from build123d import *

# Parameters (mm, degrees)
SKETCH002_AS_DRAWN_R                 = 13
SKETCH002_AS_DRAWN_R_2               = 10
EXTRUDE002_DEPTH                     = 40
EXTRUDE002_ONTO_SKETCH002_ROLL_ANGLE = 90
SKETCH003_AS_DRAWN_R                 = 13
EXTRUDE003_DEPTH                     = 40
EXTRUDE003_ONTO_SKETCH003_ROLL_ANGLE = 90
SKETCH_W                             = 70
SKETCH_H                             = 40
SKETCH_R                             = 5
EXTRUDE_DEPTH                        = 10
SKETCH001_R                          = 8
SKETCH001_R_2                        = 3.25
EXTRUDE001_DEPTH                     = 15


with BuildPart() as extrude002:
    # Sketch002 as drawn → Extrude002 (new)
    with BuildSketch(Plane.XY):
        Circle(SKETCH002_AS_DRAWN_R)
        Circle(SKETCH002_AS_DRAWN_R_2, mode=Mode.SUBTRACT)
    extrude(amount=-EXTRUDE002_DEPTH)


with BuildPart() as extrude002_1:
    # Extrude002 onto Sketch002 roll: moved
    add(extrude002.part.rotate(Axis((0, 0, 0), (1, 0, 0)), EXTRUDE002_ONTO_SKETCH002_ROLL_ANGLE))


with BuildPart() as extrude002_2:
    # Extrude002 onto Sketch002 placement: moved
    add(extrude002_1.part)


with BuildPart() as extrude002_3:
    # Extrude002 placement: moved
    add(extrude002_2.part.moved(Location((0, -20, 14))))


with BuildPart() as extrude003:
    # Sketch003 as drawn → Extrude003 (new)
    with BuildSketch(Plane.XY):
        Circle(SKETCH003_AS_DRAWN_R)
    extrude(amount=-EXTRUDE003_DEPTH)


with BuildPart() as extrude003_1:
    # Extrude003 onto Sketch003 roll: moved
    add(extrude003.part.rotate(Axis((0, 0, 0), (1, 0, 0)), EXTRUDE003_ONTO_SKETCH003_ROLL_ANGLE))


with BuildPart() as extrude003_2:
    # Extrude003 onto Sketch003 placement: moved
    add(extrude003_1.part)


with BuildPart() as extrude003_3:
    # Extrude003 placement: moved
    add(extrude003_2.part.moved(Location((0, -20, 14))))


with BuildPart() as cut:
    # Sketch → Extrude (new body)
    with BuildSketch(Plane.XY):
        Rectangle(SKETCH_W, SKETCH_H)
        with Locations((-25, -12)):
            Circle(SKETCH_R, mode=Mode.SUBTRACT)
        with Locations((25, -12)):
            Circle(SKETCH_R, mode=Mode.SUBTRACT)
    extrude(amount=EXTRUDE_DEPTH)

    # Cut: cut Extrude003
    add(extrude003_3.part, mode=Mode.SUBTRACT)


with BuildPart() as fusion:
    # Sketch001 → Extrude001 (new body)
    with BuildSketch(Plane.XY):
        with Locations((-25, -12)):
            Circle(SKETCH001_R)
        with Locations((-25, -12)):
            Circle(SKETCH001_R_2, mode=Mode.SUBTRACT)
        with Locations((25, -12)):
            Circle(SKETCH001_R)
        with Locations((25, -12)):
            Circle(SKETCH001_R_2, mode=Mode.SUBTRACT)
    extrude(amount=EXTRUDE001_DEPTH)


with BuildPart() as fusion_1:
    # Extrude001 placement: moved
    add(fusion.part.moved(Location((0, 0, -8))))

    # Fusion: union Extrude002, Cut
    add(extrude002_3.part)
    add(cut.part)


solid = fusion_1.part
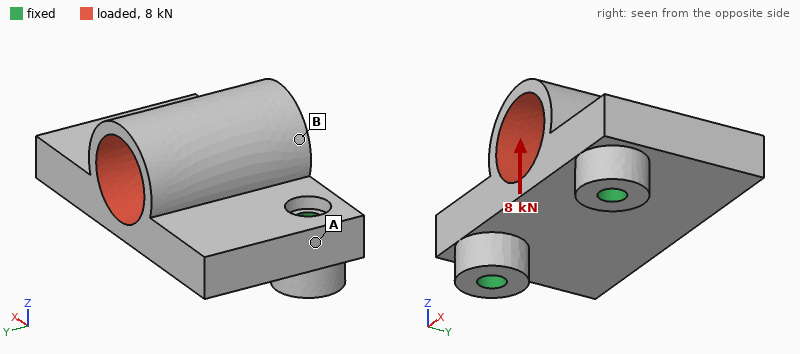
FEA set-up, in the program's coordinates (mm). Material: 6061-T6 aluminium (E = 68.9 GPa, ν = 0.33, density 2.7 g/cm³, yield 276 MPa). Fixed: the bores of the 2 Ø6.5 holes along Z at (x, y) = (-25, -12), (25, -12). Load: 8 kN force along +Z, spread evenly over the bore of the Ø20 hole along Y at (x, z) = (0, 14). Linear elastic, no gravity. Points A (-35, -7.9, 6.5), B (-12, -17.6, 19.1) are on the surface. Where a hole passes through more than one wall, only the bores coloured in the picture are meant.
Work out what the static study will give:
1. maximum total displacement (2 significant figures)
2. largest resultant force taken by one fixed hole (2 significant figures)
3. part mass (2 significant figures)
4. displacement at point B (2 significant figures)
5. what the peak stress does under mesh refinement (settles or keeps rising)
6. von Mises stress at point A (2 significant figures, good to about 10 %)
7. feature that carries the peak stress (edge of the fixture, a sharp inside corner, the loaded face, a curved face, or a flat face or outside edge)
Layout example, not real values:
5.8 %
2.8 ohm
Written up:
0.14 mm
4.0 kN
86 g
0.044 mm
keeps rising
47 MPa
edge of the fixture
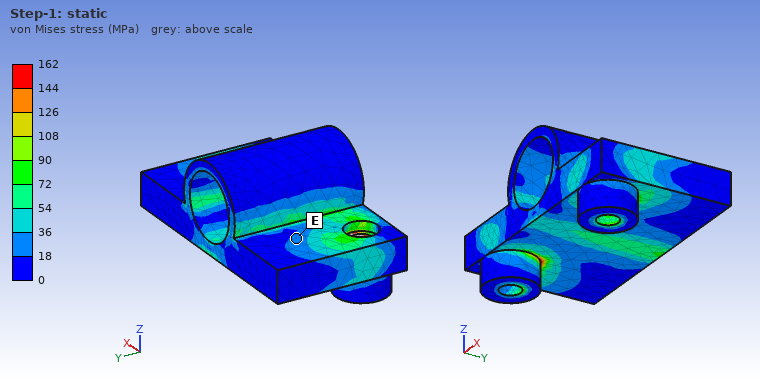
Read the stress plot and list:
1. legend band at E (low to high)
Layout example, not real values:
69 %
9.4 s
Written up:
18 to 36 MPa
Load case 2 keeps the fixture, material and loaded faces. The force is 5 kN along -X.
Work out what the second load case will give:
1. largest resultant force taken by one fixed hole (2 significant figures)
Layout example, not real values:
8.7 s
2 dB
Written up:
2.9 kN
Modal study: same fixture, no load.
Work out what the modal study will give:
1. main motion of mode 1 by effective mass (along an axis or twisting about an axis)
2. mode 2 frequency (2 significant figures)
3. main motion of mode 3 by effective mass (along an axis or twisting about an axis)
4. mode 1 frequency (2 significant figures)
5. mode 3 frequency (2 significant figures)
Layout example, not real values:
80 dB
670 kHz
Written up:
along Z
9700 Hz
along X
5600 Hz
12 kHz
